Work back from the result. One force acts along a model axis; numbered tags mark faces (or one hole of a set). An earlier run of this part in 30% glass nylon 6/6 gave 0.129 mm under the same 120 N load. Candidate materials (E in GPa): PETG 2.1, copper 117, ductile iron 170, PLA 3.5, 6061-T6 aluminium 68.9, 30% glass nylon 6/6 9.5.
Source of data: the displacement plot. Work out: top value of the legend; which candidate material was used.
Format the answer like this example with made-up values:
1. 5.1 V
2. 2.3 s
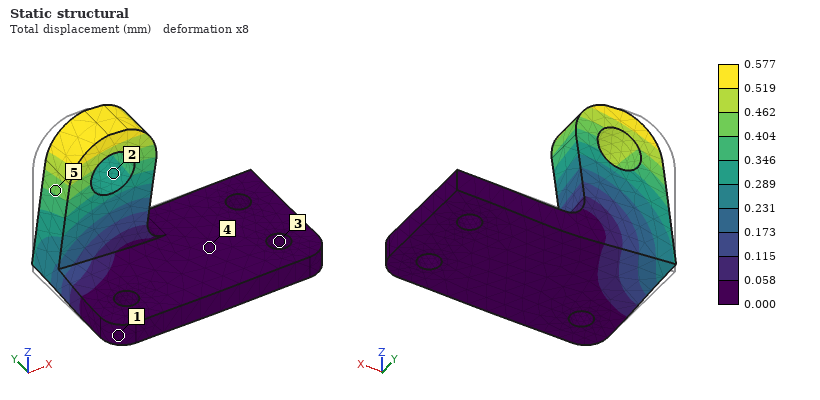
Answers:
1. 0.577 mm
2. PETG
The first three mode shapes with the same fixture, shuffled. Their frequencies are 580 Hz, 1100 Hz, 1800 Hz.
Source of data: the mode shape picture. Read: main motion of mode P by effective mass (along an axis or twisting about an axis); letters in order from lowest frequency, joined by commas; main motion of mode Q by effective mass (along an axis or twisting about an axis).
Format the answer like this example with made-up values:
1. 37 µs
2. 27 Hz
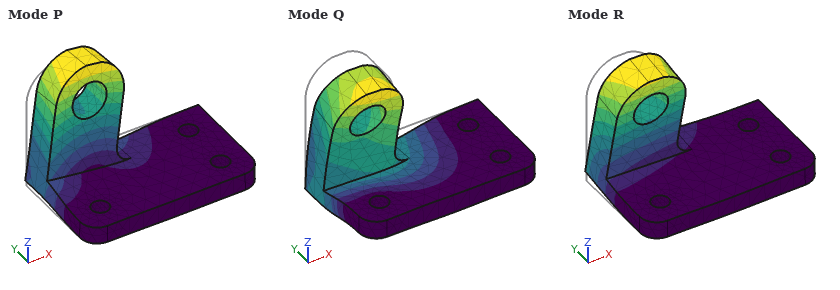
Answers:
1. along X
2. R, P, Q
3. along Z
